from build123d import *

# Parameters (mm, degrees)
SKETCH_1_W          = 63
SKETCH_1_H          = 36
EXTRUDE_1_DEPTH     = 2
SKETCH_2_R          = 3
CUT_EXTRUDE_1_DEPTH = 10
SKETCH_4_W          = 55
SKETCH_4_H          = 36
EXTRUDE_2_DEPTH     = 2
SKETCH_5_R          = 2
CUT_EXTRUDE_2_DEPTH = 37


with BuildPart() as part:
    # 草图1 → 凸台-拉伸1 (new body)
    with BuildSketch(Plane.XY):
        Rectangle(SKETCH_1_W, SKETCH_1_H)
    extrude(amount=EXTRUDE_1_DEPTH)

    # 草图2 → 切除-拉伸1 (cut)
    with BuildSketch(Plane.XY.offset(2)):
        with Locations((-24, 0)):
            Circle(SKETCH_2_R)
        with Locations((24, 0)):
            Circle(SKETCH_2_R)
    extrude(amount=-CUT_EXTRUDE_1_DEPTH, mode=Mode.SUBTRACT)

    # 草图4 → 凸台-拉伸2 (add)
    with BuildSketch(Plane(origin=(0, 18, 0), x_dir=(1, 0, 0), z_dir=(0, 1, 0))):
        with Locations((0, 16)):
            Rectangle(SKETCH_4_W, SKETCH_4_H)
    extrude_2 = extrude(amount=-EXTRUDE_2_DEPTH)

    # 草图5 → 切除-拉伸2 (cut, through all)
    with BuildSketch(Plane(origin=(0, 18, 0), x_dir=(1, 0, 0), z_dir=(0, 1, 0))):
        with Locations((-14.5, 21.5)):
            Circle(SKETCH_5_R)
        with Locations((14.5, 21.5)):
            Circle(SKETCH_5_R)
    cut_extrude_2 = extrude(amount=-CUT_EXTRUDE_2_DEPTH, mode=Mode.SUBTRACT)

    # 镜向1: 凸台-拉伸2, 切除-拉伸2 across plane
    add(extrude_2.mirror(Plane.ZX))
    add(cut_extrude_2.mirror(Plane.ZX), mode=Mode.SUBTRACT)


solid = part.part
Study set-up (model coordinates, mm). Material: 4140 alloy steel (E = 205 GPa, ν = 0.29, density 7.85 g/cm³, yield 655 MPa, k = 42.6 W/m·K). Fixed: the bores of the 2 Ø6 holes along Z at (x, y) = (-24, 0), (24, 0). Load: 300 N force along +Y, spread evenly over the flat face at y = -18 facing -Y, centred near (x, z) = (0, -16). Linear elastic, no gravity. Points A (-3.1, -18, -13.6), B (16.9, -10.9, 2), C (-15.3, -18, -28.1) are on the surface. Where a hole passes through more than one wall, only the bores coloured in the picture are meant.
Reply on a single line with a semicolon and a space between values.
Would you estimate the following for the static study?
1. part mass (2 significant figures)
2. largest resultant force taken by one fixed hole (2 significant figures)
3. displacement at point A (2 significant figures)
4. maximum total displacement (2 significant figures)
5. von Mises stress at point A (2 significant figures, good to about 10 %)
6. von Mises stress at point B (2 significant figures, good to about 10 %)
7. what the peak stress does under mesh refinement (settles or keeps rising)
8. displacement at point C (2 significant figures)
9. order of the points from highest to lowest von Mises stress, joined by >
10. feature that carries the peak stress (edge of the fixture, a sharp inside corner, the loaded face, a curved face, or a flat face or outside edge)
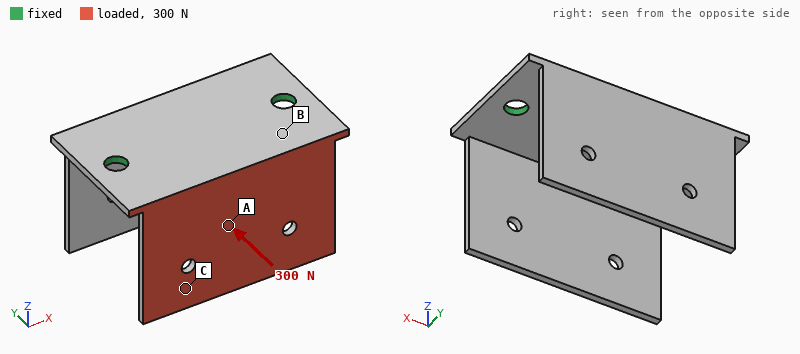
93 g; 150 N; 0.20 mm; 0.51 mm; 41 MPa; 110 MPa; keeps rising; 0.41 mm; B > A > C; edge of the fixture
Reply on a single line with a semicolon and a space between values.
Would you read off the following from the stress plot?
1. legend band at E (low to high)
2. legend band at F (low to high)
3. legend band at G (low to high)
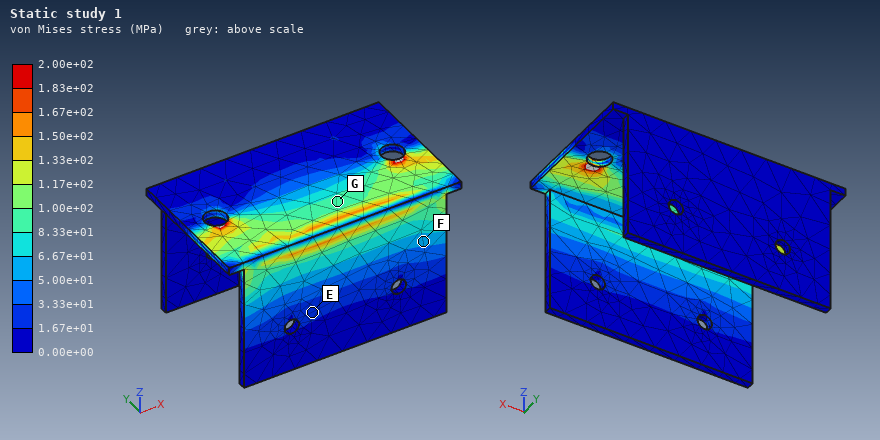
1.67e+01 to 3.33e+01 MPa; 5.00e+01 to 6.67e+01 MPa; 8.33e+01 to 1.00e+02 MPa
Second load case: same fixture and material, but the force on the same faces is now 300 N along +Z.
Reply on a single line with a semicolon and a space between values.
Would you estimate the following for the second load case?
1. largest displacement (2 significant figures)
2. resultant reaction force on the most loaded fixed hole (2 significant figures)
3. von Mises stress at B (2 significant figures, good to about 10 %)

0.20 mm; 150 N; 53 MPa
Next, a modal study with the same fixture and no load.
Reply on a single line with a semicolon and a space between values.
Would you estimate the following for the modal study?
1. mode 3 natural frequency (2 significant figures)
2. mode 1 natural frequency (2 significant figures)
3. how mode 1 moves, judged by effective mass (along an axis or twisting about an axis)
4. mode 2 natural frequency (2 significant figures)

1800 Hz; 810 Hz; along Y; 850 Hz
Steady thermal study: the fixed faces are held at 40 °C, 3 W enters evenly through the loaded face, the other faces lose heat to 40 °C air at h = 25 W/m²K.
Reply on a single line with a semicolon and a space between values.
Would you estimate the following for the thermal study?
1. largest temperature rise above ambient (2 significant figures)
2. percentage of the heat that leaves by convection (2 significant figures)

16 K; 39 %
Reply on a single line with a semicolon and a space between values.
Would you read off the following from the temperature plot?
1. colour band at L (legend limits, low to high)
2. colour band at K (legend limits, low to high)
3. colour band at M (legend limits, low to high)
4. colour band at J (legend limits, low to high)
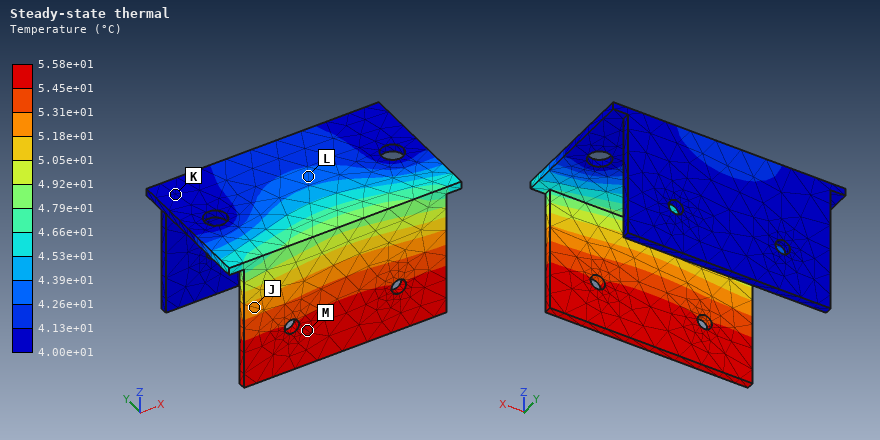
4.26e+01 to 4.39e+01 °C; 4.00e+01 to 4.13e+01 °C; 5.45e+01 to 5.58e+01 °C; 5.18e+01 to 5.31e+01 °C
